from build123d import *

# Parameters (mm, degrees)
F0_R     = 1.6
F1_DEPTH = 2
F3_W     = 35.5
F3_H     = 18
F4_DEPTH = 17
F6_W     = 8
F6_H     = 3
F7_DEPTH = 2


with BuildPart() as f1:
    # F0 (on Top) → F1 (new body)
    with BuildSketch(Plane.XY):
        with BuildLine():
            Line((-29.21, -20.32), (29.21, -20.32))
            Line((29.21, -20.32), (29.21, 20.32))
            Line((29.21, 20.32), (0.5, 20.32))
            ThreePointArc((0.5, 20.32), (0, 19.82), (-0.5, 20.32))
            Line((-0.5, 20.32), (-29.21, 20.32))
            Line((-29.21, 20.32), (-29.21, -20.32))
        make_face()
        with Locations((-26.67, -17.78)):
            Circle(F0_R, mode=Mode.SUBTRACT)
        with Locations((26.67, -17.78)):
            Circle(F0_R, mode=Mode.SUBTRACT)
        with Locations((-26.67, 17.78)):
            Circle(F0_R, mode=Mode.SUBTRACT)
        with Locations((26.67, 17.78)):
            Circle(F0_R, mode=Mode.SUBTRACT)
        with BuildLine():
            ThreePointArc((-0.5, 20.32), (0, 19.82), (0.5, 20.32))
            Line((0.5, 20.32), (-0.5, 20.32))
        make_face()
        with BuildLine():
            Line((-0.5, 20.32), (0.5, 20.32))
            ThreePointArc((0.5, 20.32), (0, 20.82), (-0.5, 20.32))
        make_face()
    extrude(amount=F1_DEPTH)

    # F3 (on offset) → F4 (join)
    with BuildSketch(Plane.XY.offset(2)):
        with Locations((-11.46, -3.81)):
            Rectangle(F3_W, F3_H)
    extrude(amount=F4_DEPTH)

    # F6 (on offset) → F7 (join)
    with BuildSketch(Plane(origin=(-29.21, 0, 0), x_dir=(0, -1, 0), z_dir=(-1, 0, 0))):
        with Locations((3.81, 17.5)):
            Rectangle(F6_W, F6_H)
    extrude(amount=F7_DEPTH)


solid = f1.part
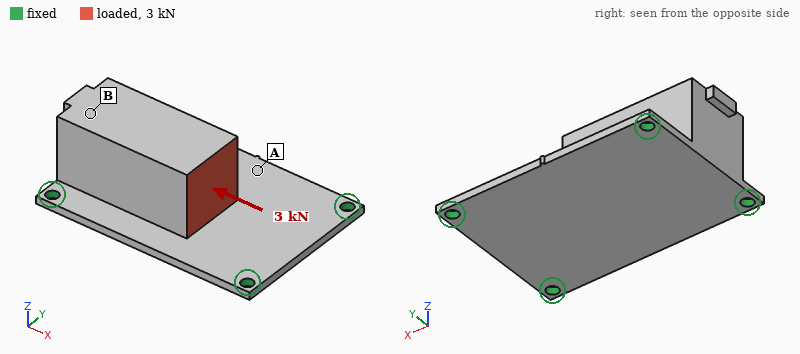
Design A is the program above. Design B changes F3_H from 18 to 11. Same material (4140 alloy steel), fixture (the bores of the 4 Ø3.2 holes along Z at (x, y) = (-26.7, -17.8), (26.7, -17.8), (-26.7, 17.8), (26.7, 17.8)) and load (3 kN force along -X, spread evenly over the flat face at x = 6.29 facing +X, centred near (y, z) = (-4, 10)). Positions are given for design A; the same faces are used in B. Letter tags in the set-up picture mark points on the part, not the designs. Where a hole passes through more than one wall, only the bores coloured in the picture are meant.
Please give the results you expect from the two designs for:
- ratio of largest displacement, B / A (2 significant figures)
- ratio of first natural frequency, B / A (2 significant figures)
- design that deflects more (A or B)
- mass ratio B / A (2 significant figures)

1.2
1.1
B
0.73
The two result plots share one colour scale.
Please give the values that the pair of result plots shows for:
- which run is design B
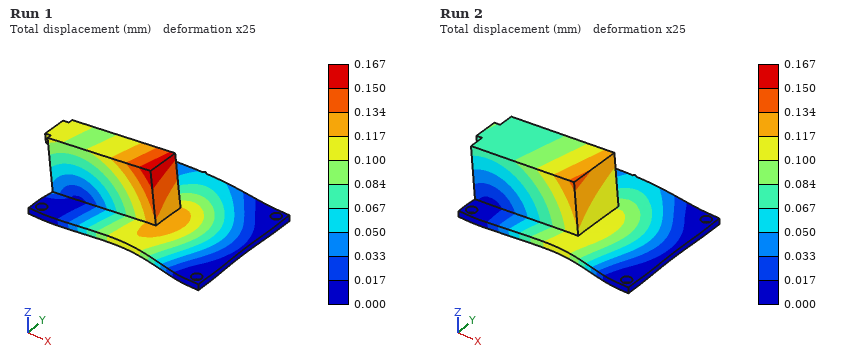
Run 1
